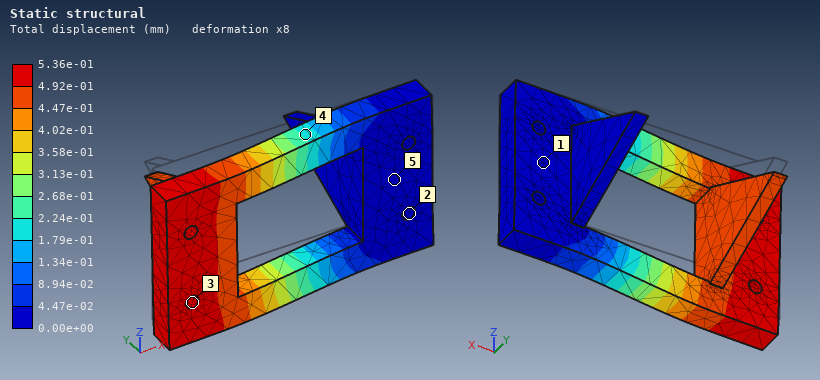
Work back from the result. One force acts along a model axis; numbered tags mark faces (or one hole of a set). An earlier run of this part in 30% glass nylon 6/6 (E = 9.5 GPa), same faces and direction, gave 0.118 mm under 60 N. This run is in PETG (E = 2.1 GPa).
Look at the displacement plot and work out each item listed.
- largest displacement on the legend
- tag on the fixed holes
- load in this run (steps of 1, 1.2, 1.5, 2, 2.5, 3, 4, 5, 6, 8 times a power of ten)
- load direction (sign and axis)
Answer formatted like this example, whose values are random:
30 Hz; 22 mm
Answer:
5.36e-01 mm; 2; 60 N; -Z
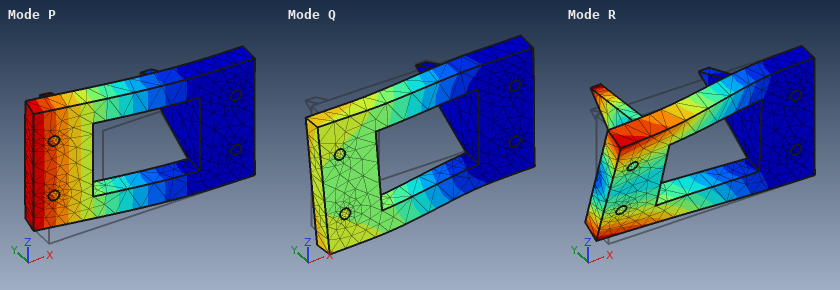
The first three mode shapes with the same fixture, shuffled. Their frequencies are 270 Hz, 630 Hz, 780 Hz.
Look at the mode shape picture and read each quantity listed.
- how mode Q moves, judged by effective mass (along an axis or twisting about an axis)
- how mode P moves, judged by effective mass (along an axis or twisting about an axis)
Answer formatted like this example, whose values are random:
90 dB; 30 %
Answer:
along Z; along Y
